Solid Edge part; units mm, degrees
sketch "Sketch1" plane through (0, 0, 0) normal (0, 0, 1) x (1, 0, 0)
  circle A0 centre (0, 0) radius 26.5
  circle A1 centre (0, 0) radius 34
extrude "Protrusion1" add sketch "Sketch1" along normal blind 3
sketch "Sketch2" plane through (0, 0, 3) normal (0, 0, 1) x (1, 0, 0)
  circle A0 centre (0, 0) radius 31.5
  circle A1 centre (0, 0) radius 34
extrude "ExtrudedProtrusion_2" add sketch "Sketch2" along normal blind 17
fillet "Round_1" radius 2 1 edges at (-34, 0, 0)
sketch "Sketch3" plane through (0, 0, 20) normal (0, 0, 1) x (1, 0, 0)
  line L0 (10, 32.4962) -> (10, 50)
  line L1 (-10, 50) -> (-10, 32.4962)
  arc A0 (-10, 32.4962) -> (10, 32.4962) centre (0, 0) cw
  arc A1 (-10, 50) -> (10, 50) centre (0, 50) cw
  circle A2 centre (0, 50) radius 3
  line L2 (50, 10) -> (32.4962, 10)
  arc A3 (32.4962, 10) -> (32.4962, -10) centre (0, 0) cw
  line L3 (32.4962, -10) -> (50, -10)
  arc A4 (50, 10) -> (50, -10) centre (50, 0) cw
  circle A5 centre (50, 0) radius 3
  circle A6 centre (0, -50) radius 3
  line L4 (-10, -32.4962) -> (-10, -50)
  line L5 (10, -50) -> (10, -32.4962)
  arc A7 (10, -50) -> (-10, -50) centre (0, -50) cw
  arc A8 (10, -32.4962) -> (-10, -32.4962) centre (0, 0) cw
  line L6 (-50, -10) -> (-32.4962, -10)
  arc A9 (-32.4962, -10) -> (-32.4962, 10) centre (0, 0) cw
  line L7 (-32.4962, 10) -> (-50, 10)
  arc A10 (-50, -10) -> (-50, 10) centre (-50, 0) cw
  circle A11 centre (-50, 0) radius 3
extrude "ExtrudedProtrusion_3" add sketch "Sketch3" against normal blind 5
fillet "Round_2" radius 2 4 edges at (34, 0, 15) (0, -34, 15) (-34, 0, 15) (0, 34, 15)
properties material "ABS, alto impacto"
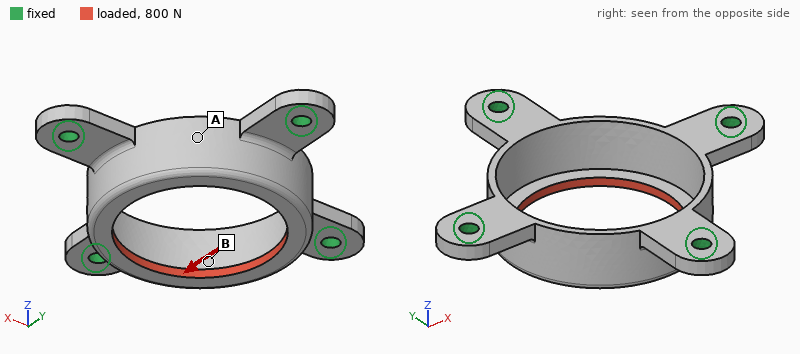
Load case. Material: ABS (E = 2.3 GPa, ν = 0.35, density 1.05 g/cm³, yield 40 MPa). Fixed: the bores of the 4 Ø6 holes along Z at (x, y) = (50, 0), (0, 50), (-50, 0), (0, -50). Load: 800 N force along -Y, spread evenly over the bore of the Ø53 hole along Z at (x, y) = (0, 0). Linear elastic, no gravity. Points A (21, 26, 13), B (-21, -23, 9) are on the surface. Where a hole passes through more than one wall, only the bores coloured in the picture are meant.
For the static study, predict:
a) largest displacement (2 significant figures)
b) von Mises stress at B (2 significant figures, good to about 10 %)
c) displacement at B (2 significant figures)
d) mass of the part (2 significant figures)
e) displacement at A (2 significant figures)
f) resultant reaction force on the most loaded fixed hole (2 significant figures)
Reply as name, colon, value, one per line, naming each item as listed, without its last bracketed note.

largest displacement: 0.39 mm
von Mises stress at B: 6.1 MPa
displacement at B: 0.27 mm
mass of the part: 23 g
displacement at A: 0.25 mm
resultant reaction force on the most loaded fixed hole: 240 N
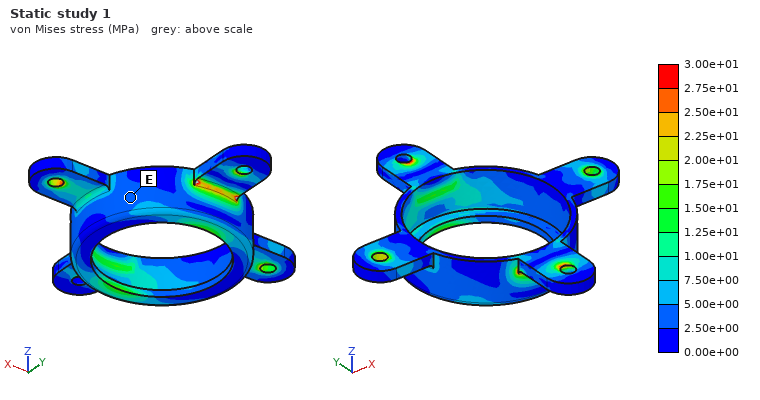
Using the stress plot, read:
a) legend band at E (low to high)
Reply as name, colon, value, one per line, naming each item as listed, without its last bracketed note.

legend band at E: 2.50e+00 to 5.00e+00 MPa
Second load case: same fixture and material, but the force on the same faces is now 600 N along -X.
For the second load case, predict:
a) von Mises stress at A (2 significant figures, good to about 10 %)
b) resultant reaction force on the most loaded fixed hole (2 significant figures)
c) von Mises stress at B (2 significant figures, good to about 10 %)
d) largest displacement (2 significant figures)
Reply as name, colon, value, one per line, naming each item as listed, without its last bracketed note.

von Mises stress at A: 2.0 MPa
resultant reaction force on the most loaded fixed hole: 180 N
von Mises stress at B: 4.1 MPa
largest displacement: 0.29 mm
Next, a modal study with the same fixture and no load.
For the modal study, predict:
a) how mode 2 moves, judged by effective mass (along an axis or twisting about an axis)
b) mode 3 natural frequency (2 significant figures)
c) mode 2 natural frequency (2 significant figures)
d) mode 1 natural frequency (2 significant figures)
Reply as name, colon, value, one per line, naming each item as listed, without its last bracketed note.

how mode 2 moves, judged by effective mass: along Z
mode 3 natural frequency: 2000 Hz
mode 2 natural frequency: 1900 Hz
mode 1 natural frequency: 1700 Hz
